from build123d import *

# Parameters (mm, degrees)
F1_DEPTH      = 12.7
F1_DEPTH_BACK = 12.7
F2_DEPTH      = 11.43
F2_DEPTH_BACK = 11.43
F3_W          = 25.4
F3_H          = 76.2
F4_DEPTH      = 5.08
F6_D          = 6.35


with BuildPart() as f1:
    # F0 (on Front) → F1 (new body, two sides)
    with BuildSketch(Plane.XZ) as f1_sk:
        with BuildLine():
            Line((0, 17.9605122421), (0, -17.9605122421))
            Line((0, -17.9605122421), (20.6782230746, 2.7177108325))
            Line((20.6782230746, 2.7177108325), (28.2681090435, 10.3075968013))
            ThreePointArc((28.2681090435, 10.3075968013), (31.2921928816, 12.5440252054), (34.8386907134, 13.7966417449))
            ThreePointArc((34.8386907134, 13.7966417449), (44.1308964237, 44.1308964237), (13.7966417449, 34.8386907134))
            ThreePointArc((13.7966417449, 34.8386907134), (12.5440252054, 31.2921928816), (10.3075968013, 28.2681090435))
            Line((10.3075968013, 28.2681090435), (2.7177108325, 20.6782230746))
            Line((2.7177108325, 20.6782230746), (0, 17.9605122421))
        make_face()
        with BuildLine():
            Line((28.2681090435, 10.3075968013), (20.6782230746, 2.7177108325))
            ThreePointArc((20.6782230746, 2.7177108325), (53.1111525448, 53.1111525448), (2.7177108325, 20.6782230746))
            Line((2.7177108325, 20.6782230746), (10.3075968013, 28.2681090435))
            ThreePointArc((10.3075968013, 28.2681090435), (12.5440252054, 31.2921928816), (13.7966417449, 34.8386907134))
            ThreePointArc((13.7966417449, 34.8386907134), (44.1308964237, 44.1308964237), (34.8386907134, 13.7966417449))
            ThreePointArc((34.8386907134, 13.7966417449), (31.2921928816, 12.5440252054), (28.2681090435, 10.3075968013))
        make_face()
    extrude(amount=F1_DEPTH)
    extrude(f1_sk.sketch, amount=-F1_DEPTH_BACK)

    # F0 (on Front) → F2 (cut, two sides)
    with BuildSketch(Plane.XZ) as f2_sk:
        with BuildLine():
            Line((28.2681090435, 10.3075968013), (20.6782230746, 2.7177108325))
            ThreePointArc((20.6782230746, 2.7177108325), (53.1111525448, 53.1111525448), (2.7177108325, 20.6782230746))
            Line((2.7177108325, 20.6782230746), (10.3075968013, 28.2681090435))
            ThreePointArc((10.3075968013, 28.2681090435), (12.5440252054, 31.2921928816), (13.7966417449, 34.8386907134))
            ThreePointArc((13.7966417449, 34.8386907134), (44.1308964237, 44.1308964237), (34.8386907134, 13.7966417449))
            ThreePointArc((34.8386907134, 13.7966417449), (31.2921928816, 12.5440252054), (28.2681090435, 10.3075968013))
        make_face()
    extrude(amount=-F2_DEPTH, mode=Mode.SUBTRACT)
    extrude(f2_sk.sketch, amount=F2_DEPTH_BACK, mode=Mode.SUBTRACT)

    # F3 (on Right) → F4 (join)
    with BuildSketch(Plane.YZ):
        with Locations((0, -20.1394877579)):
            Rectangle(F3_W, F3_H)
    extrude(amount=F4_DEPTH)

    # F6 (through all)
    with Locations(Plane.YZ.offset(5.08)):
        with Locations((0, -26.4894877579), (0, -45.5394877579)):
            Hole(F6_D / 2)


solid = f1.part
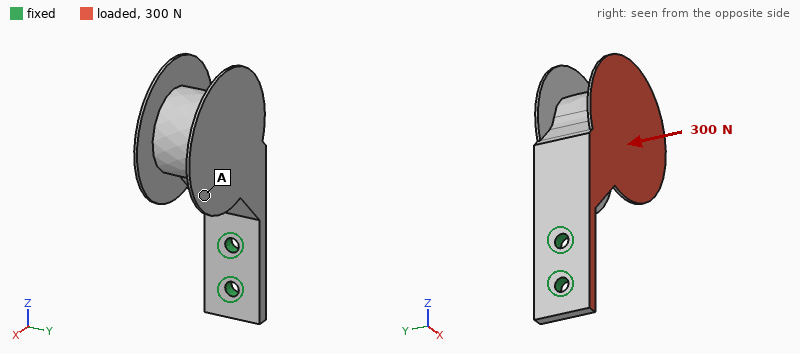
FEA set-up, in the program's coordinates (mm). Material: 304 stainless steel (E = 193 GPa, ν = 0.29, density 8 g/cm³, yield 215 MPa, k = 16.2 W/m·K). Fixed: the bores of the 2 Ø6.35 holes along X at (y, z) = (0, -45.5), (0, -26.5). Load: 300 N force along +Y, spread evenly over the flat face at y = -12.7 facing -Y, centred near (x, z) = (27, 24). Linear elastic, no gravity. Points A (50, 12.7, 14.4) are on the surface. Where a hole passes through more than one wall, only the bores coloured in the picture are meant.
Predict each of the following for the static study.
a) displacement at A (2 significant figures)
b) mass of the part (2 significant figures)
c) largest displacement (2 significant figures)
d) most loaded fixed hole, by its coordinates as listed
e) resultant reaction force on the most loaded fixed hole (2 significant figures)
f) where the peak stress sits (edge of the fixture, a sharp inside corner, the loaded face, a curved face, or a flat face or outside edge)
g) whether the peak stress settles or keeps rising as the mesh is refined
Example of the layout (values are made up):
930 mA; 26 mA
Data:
63 µm; 430 g; 89 µm; (0, -26.5); 750 N; edge of the fixture; keeps rising
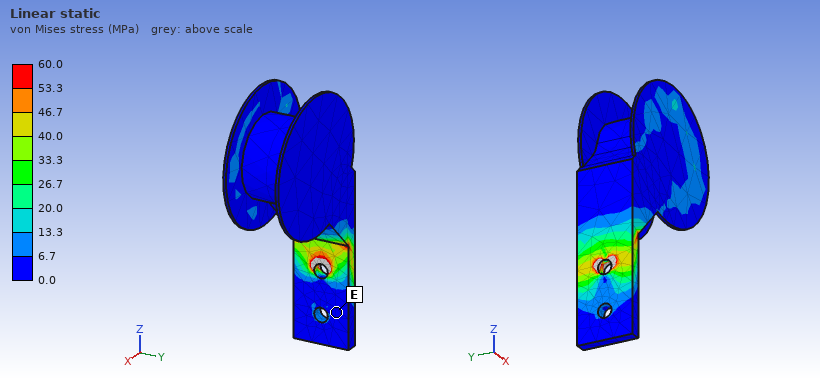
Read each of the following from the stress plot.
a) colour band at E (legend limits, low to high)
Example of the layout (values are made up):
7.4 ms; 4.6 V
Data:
0.0 to 6.7 MPa
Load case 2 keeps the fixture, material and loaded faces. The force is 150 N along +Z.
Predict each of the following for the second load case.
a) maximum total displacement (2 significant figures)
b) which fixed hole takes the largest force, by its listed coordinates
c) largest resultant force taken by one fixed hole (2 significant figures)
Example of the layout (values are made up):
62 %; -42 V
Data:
95 µm; (0, -26.5); 140 N
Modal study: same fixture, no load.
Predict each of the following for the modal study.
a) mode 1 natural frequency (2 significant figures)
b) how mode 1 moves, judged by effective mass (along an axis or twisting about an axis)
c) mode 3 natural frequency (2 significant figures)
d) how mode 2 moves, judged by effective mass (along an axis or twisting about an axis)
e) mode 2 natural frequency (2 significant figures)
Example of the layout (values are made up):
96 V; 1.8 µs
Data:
300 Hz; along X; 2200 Hz; along Y; 690 Hz
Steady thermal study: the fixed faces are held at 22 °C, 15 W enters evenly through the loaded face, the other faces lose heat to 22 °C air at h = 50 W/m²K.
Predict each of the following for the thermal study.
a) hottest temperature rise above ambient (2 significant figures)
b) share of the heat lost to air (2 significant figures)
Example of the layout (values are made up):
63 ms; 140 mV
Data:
41 K; 84 %
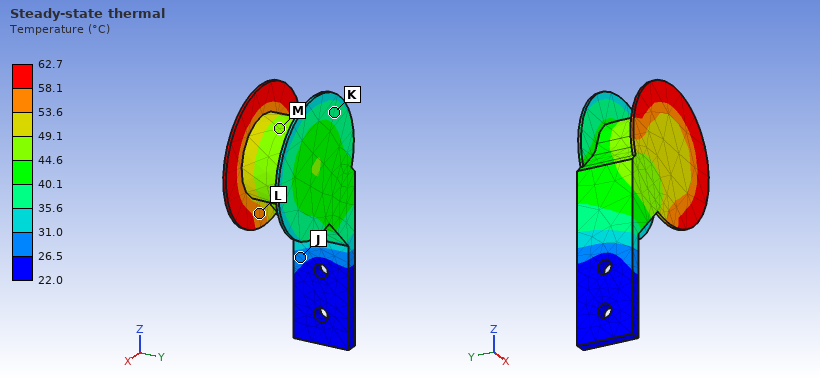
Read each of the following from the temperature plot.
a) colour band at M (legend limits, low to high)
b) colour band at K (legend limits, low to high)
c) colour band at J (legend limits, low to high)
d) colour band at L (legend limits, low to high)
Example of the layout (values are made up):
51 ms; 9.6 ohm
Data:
44.6 to 49.1 °C; 35.6 to 40.1 °C; 26.5 to 31.0 °C; 53.6 to 58.1 °C
